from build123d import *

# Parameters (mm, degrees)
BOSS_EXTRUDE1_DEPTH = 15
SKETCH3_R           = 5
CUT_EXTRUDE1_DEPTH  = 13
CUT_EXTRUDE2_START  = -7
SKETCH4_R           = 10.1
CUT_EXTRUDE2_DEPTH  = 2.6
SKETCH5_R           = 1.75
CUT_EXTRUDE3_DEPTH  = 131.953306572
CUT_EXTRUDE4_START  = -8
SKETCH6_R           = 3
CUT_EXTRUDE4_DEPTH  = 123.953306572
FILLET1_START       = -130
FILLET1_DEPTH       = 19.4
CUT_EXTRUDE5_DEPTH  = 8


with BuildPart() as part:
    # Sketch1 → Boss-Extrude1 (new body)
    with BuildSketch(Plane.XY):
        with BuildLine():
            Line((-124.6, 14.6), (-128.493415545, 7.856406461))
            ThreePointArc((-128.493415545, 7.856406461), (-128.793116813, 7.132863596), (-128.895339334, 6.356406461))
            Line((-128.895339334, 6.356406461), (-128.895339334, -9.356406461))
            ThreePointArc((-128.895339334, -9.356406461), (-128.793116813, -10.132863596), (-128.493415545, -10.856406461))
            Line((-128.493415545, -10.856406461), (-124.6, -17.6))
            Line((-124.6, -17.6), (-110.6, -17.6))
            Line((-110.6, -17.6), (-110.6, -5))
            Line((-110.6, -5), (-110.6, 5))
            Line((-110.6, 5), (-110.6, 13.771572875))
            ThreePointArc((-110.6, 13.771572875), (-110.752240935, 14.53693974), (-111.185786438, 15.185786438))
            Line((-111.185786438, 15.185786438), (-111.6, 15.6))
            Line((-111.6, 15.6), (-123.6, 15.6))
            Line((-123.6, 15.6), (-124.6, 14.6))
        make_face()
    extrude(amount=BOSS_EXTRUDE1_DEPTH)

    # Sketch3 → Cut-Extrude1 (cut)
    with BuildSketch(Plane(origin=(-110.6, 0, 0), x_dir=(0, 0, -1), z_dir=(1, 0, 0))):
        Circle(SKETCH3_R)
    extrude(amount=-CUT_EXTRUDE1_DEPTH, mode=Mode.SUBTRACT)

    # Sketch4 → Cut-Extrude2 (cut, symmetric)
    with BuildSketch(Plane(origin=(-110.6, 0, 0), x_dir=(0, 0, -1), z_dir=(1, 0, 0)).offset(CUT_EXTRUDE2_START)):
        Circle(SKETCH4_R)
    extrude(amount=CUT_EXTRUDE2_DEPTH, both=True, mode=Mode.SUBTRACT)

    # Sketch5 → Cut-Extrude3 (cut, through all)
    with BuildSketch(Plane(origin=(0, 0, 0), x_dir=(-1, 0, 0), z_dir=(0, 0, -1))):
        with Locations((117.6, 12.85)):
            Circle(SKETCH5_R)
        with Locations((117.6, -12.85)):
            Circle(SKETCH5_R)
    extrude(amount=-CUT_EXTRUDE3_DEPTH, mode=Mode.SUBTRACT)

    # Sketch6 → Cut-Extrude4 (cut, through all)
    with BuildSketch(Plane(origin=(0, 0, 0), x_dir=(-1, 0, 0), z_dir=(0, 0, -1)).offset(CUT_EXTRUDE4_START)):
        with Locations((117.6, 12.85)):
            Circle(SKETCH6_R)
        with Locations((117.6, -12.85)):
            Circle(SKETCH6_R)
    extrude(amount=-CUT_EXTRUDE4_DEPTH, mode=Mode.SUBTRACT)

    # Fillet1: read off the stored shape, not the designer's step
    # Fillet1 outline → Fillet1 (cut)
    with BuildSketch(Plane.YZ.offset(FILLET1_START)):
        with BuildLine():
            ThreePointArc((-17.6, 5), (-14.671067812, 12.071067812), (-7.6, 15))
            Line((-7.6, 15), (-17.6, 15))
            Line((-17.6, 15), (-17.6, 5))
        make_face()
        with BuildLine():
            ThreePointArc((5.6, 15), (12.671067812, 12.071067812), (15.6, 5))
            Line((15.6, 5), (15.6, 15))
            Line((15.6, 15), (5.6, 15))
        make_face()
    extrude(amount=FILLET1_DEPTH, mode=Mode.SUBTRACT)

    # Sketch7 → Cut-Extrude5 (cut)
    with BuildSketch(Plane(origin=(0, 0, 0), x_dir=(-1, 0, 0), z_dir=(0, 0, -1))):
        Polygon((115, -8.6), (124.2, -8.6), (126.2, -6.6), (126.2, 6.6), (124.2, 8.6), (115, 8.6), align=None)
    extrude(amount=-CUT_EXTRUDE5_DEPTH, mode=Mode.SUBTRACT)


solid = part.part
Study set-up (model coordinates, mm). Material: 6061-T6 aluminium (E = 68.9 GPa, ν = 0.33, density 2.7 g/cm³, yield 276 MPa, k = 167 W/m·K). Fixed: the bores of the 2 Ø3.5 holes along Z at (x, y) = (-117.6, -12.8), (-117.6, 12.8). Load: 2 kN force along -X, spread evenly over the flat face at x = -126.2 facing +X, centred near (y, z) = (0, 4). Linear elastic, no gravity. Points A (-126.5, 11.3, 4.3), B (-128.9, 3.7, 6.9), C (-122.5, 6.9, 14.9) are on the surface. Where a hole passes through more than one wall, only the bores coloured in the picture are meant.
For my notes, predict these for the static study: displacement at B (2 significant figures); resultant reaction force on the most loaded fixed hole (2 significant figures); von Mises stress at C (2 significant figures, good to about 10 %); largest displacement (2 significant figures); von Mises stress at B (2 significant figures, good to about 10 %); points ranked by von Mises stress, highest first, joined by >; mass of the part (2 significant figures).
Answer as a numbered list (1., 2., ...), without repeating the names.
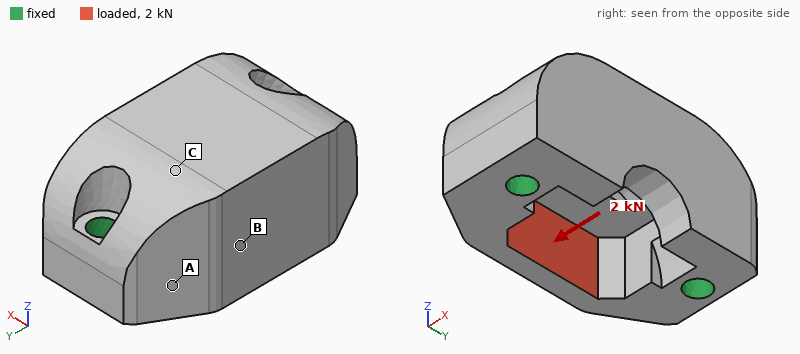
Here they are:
1. 14 µm
2. 1.1 kN
3. 13 MPa
4. 48 µm
5. 84 MPa
6. B > A > C
7. 15 g
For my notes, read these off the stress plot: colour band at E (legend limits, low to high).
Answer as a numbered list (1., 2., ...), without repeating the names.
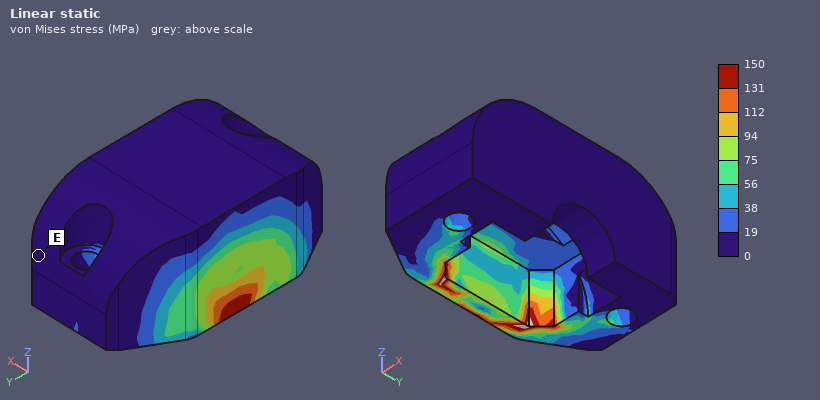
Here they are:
1. 0 to 19 MPa
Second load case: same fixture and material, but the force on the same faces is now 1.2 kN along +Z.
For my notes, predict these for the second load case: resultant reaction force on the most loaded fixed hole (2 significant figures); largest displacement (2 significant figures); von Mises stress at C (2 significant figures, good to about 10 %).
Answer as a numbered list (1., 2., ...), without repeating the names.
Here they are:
1. 650 N
2. 16 µm
3. 13 MPa
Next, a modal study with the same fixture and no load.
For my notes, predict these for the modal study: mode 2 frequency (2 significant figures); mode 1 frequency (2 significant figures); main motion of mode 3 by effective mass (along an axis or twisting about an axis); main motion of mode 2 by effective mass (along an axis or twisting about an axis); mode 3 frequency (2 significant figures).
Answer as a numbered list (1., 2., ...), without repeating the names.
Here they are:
1. 33 kHz
2. 21 kHz
3. along Z
4. along Y
5. 36 kHz
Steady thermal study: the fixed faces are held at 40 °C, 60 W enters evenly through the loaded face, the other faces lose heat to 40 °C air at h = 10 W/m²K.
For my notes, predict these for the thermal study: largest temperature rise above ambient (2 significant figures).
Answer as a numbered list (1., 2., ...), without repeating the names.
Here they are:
1. 51 K
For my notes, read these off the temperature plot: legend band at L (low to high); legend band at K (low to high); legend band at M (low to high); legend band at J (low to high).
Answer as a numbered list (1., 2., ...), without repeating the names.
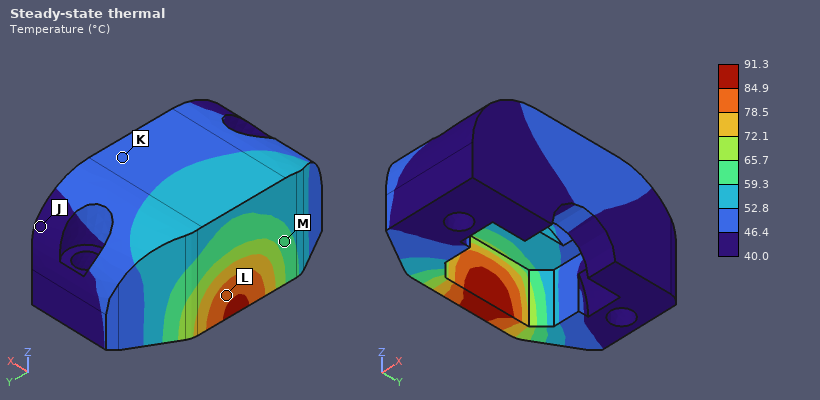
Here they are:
1. 78.5 to 84.9 °C
2. 46.4 to 52.8 °C
3. 59.3 to 65.7 °C
4. 40.0 to 46.4 °C
